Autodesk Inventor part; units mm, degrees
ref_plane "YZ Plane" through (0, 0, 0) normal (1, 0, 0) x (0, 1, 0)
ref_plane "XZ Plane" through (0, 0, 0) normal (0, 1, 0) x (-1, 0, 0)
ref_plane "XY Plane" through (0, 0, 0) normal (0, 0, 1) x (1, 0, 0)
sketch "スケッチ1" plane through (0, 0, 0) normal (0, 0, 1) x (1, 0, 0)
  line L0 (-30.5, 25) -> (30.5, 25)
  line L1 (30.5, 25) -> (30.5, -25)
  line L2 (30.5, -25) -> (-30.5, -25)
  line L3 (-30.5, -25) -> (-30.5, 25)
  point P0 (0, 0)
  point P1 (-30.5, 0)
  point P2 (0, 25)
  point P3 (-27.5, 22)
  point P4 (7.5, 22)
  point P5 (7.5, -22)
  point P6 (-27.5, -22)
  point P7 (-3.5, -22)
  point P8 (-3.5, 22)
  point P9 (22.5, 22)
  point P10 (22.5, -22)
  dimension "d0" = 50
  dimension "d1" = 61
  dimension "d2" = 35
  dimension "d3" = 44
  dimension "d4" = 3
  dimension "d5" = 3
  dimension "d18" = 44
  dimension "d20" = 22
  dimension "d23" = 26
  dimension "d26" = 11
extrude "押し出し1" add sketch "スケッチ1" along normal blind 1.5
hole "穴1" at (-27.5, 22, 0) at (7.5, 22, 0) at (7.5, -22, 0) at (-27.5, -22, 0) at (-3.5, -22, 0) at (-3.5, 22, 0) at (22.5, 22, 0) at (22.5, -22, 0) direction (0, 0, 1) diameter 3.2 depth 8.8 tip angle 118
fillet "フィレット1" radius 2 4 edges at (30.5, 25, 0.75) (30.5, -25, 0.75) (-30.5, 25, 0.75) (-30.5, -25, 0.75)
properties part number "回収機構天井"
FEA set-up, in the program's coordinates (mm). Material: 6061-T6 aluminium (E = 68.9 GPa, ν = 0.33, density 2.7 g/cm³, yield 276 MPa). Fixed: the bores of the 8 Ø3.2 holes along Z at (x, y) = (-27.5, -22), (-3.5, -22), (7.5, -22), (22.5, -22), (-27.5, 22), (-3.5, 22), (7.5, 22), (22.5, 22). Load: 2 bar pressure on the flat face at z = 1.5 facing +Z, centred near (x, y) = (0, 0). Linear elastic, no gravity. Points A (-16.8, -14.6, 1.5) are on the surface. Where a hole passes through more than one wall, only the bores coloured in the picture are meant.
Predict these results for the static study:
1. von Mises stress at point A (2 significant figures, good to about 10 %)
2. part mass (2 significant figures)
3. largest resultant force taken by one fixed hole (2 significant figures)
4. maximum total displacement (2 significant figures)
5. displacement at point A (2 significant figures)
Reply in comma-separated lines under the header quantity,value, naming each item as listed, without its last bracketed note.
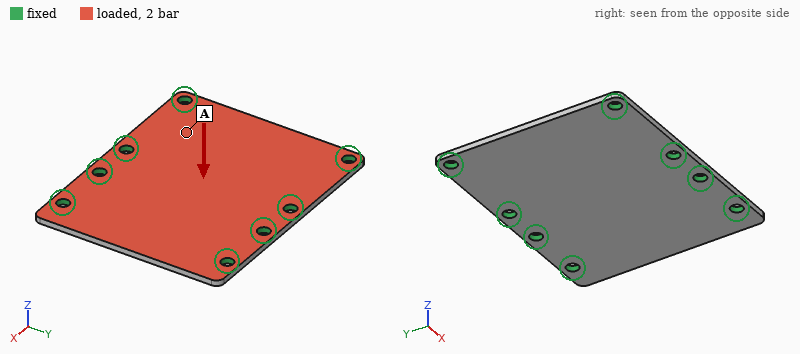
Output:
quantity,value
von Mises stress at point A,18 MPa
part mass,12 g
largest resultant force taken by one fixed hole,88 N
maximum total displacement,0.11 mm
displacement at point A,0.046 mm
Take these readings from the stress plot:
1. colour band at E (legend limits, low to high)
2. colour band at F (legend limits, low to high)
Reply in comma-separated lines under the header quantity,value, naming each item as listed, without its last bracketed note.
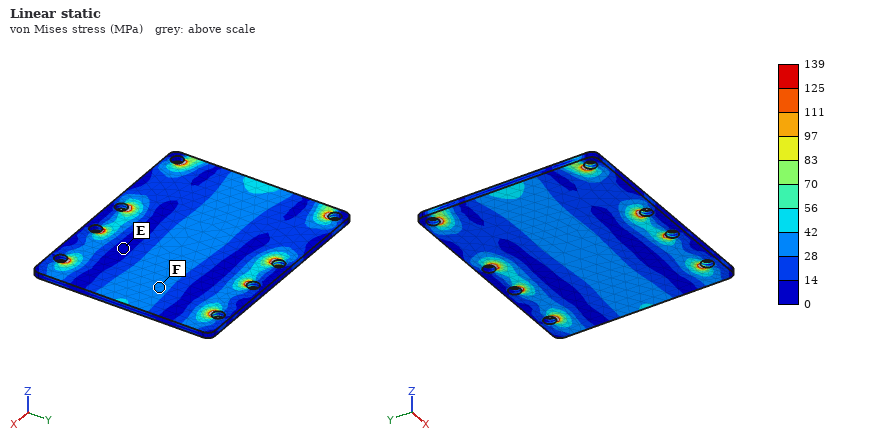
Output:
quantity,value
colour band at E,0 to 14 MPa
colour band at F,28 to 42 MPa
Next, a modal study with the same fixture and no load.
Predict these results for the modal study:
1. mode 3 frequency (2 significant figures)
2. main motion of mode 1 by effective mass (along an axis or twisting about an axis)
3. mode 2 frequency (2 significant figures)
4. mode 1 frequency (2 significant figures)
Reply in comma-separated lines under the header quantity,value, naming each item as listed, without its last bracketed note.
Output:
quantity,value
mode 3 frequency,6300 Hz
main motion of mode 1 by effective mass,along Z
mode 2 frequency,4500 Hz
mode 1 frequency,4100 Hz
